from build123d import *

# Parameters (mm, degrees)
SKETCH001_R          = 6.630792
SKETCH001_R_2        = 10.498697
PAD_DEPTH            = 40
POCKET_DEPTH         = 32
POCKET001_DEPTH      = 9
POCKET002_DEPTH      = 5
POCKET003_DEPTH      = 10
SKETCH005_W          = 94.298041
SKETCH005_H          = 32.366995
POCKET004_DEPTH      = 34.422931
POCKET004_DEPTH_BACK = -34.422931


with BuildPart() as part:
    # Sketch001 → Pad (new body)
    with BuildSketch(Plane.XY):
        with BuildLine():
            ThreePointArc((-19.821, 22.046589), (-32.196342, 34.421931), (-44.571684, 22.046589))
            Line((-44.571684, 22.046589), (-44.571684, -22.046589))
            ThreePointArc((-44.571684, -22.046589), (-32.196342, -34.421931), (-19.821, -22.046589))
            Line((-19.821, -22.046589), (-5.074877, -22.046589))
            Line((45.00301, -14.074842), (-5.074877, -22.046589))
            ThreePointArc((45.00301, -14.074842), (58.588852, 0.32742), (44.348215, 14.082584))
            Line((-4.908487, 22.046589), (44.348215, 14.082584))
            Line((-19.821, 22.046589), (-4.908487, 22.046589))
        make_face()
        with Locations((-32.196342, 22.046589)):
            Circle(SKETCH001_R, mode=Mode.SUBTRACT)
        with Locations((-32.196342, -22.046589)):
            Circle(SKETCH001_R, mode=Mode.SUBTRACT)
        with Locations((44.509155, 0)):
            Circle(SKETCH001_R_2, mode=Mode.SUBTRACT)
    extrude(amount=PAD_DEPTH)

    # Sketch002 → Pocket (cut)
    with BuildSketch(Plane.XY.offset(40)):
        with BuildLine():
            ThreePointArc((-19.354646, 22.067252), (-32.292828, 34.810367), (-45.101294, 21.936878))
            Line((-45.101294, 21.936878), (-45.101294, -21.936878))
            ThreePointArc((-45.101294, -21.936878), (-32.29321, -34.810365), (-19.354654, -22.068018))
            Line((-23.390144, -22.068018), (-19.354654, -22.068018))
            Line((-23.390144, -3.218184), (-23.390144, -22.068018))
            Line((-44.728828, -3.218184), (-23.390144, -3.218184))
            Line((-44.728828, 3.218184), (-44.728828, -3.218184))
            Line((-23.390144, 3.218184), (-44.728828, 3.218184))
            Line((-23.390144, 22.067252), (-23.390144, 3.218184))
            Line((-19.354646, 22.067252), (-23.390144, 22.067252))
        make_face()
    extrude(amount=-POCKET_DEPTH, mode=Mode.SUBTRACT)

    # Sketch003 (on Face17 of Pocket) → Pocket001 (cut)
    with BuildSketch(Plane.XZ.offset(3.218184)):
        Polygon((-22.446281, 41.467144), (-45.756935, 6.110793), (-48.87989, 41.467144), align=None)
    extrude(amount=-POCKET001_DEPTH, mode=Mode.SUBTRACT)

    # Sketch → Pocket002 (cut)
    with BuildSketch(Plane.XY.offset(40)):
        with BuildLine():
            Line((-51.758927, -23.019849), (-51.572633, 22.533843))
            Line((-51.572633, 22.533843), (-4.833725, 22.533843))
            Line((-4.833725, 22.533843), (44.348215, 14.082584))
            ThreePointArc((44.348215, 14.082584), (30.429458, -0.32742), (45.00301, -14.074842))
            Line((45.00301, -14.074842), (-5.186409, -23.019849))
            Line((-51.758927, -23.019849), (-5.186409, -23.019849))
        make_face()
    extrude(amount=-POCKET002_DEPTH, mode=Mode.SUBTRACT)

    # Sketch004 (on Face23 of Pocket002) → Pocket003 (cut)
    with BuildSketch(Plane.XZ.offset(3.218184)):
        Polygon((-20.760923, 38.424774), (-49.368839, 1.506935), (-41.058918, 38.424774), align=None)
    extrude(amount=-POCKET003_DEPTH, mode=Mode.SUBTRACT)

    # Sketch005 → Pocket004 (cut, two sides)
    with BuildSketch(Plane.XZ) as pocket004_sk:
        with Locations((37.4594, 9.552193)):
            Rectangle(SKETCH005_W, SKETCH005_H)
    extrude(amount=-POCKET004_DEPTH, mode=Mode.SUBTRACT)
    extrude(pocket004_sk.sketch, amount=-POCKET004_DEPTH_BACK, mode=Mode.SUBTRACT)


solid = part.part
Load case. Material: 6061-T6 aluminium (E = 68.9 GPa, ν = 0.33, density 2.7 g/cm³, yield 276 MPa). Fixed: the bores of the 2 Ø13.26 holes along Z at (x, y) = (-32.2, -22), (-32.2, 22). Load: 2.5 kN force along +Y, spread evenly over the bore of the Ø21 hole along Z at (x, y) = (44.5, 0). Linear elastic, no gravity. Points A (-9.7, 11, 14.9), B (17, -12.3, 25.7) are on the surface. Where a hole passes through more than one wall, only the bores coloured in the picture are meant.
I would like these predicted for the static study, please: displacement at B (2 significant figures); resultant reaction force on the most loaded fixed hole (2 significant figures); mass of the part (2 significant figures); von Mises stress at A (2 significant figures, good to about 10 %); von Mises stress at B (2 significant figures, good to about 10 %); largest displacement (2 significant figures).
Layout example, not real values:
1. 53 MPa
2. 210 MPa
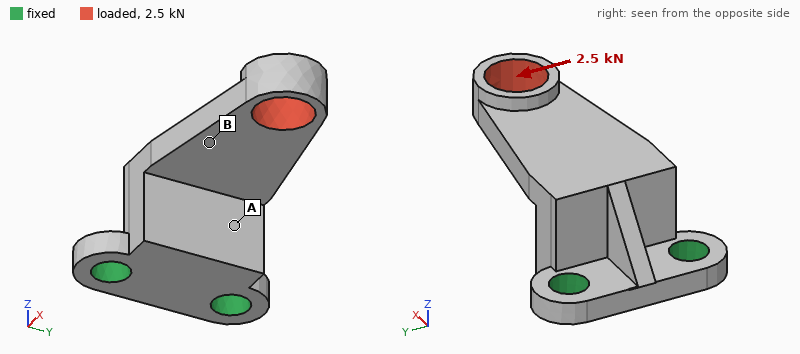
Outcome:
1. 0.15 mm
2. 4.8 kN
3. 140 g
4. 79 MPa
5. 24 MPa
6. 0.38 mm
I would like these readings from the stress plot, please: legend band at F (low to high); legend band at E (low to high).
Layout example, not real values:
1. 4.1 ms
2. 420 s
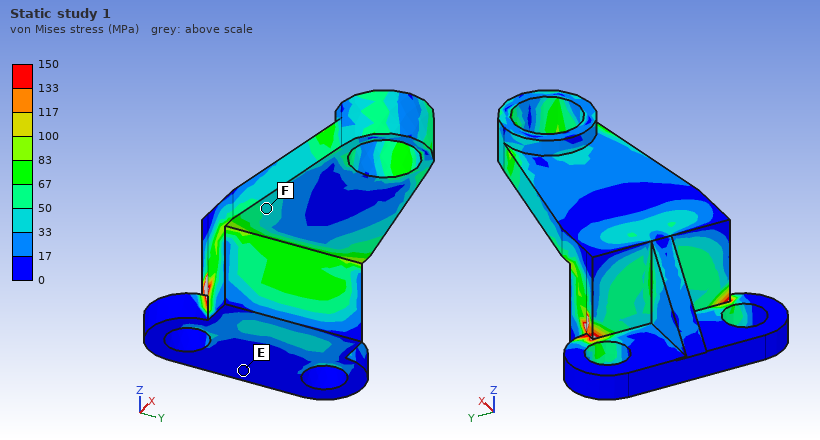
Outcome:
1. 33 to 50 MPa
2. 0 to 17 MPa
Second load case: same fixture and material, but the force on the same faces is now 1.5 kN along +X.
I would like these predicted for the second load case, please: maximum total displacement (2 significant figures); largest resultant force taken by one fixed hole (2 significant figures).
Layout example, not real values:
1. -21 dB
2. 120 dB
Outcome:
1. 0.23 mm
2. 750 N
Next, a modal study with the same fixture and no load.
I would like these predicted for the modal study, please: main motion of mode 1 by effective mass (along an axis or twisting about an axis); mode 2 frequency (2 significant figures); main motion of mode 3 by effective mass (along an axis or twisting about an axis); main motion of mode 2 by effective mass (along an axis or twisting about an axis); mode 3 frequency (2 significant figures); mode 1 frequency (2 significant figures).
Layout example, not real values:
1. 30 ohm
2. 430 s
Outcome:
1. along Z
2. 3200 Hz
3. along X
4. along Y
5. 4100 Hz
6. 1400 Hz
